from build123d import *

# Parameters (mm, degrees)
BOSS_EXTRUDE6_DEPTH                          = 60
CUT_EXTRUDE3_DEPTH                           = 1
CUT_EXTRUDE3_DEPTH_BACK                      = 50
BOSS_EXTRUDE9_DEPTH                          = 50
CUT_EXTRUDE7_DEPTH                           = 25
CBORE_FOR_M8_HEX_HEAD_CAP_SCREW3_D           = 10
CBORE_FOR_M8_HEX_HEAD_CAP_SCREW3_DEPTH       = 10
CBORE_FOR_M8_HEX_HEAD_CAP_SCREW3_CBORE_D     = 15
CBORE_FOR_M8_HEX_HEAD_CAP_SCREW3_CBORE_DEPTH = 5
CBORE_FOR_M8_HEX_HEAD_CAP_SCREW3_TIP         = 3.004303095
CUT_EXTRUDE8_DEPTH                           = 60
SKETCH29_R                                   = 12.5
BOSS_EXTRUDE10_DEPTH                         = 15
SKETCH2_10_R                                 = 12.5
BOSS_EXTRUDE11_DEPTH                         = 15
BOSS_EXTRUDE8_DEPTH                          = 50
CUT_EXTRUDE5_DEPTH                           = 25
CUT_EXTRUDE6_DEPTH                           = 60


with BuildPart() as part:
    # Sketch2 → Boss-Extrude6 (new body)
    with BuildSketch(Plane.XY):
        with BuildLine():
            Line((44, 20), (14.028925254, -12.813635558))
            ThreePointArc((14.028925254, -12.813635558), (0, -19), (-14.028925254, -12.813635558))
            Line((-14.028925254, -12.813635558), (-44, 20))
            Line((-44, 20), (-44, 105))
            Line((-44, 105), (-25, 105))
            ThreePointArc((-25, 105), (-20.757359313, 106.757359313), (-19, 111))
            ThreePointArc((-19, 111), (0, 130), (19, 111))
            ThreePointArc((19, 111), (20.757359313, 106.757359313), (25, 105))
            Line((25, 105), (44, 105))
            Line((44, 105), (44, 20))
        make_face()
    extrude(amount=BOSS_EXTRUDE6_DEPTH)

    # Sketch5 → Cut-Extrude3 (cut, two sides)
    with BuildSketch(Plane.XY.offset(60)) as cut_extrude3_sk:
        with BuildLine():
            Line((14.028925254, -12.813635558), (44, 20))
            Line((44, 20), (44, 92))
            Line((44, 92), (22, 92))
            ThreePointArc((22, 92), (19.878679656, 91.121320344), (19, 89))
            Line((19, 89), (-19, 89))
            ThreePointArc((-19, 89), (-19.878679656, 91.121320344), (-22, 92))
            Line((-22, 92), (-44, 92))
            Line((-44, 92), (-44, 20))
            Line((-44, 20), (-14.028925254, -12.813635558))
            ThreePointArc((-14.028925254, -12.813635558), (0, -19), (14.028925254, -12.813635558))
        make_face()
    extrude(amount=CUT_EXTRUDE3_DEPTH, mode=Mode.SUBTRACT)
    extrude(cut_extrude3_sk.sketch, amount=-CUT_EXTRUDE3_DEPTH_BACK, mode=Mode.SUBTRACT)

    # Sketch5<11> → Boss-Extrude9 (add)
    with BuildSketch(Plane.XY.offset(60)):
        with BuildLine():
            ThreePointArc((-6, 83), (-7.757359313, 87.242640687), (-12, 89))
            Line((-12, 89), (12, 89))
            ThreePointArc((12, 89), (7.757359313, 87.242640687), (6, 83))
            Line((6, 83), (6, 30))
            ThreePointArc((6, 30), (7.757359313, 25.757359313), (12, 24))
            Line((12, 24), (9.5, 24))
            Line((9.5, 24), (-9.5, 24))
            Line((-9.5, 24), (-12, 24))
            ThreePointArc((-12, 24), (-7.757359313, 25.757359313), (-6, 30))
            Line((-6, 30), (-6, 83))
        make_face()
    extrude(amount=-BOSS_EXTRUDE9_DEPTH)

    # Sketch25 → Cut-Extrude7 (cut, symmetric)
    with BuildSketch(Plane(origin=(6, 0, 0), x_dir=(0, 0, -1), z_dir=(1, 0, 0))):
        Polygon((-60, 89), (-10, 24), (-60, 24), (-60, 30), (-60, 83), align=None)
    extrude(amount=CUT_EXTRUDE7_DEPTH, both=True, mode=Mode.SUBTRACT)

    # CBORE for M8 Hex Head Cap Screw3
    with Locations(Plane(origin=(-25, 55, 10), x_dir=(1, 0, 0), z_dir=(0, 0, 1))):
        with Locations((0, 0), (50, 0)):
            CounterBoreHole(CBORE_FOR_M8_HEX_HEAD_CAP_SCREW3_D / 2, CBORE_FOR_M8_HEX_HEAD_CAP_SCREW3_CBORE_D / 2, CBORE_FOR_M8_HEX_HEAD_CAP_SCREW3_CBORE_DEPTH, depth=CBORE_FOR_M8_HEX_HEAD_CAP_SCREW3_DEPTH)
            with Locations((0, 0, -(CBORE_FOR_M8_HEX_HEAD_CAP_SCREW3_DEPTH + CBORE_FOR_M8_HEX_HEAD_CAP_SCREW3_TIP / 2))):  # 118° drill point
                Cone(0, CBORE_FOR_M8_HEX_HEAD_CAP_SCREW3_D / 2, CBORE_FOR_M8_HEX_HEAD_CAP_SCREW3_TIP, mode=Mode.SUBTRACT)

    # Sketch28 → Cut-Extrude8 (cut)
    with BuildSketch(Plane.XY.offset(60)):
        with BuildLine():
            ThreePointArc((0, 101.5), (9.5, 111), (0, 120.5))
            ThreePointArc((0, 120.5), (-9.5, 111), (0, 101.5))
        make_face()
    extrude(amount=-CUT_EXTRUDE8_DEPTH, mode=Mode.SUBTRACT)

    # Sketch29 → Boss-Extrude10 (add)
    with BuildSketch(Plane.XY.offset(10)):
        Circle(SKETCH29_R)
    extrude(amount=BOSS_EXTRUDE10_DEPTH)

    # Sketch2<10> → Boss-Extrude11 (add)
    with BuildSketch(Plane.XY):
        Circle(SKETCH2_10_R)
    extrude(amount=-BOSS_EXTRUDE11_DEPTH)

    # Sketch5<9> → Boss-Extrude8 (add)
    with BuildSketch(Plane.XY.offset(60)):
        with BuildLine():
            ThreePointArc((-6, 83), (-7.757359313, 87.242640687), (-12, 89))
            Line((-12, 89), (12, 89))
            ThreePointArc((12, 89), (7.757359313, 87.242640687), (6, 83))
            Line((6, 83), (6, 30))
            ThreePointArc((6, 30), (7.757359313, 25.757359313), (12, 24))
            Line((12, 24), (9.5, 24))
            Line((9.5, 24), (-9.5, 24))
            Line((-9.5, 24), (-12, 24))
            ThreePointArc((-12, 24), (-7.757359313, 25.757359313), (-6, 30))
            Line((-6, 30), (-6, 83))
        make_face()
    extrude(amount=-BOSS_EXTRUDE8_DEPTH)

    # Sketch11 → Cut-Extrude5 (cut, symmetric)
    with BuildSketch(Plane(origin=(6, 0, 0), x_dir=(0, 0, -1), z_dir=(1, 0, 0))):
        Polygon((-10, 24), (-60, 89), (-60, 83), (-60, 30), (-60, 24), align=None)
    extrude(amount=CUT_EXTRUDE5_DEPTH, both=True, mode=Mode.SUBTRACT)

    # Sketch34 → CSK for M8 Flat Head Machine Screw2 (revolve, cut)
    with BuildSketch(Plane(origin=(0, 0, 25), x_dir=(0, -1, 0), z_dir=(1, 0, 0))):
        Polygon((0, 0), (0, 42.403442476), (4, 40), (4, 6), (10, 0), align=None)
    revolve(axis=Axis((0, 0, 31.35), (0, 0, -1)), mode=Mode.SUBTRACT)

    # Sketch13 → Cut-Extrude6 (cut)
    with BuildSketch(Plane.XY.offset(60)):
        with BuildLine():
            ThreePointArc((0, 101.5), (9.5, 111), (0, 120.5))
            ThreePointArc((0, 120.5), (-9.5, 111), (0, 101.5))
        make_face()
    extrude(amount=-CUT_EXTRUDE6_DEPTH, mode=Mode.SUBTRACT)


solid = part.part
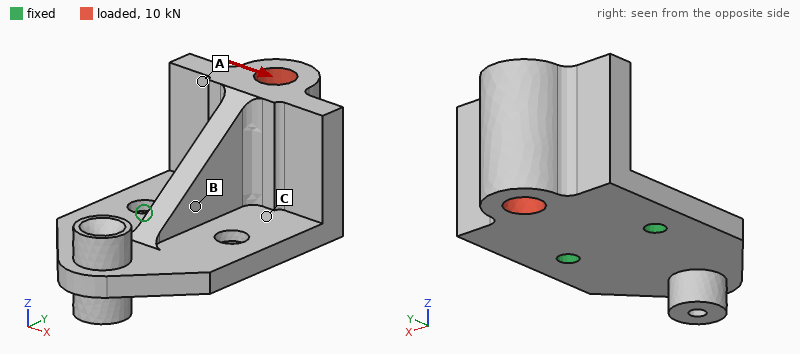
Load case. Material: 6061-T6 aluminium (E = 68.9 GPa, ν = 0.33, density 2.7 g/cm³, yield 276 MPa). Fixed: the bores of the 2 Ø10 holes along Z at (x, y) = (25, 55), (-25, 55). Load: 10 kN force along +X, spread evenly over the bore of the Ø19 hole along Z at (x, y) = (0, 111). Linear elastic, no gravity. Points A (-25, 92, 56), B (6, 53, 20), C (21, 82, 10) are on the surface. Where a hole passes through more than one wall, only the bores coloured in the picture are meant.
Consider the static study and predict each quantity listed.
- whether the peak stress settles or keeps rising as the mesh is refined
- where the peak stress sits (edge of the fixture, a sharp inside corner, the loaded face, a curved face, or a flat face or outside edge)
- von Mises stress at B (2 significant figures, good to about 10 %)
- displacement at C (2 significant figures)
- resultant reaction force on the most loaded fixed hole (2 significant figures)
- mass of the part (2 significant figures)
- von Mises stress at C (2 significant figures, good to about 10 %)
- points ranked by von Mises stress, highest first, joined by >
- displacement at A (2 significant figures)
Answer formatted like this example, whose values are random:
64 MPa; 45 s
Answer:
keeps rising; edge of the fixture; 44 MPa; 0.061 mm; 13 kN; 590 g; 70 MPa; C > B > A; 0.22 mm
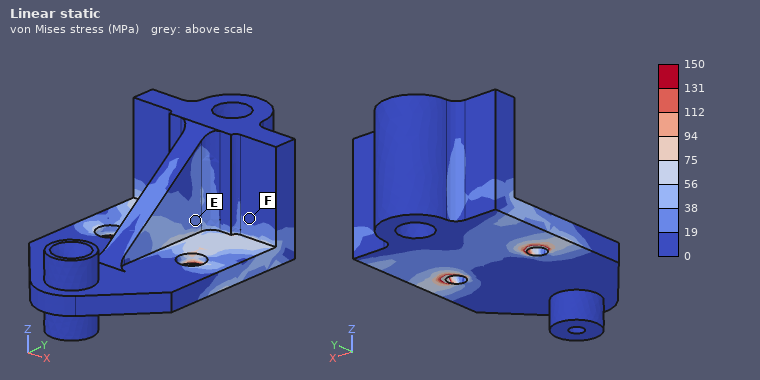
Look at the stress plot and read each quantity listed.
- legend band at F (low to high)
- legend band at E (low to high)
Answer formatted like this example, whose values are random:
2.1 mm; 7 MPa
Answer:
0 to 19 MPa; 19 to 38 MPa
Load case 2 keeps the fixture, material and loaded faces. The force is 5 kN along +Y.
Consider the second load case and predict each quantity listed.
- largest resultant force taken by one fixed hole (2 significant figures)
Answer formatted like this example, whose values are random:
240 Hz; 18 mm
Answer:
2.5 kN
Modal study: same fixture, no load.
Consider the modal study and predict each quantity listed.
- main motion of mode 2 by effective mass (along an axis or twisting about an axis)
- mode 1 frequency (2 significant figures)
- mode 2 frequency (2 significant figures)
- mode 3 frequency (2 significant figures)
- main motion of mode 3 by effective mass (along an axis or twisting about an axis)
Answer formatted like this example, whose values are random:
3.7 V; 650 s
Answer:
along X; 730 Hz; 1900 Hz; 2100 Hz; along Z
